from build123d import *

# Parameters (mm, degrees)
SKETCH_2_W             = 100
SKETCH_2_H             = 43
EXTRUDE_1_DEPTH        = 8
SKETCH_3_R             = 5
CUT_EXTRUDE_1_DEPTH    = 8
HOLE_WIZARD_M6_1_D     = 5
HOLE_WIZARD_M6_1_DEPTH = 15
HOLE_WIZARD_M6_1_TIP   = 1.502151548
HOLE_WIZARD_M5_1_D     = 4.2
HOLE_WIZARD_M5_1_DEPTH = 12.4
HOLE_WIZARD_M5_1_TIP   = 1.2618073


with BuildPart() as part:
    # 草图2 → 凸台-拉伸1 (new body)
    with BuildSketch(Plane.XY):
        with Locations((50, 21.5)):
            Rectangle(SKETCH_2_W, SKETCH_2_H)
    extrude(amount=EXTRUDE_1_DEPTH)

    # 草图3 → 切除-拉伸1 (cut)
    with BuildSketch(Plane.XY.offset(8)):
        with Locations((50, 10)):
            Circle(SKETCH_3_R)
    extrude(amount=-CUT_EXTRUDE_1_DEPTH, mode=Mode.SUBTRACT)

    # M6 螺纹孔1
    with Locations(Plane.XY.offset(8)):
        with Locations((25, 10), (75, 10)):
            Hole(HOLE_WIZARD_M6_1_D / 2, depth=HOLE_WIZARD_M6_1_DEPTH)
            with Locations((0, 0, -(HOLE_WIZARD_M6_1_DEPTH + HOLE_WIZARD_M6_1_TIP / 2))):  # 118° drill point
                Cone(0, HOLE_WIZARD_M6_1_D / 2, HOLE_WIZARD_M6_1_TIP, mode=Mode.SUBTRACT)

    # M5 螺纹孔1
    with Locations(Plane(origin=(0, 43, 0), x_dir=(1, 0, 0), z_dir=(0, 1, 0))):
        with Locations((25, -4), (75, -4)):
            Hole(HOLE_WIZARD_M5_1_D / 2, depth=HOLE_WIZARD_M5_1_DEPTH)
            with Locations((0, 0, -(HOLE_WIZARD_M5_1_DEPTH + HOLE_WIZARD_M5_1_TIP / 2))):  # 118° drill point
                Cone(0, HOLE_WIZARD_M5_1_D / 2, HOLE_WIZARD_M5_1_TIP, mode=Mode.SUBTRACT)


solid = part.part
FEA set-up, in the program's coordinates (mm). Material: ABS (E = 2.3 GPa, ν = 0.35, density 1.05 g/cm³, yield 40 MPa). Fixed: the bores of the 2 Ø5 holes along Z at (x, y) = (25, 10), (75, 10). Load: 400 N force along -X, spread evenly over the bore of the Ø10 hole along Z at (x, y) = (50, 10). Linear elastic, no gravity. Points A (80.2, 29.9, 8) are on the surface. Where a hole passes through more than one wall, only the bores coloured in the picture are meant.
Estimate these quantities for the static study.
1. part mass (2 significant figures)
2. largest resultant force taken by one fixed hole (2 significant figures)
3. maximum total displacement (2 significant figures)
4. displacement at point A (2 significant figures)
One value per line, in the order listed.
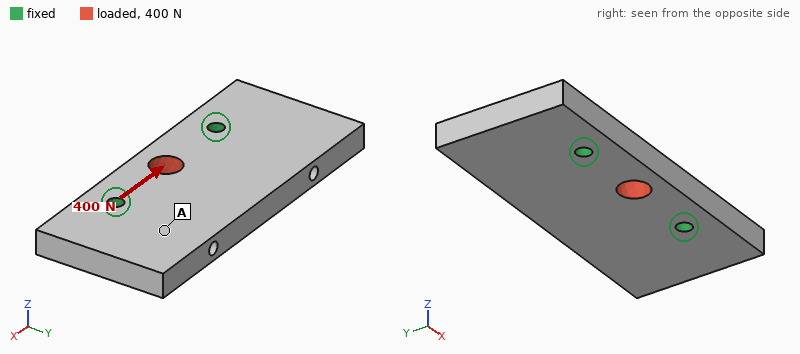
35 g
200 N
16 µm
6.2 µm
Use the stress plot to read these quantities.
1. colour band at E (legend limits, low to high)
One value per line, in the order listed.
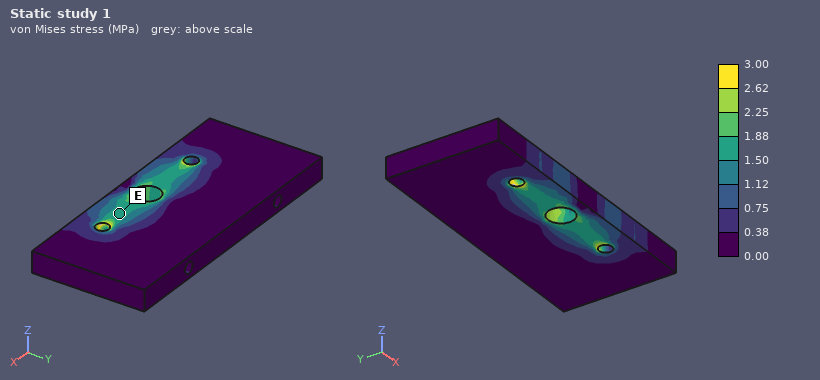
1.50 to 1.88 MPa
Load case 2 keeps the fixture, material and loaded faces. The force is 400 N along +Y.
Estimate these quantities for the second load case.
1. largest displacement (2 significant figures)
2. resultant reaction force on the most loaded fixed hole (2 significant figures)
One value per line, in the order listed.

43 µm
210 N
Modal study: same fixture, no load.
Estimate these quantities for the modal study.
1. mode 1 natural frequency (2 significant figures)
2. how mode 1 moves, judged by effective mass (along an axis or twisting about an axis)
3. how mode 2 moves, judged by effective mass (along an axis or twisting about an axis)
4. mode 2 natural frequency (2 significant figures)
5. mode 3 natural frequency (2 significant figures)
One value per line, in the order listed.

1300 Hz
along Z
twisting about Y
1500 Hz
2000 Hz
